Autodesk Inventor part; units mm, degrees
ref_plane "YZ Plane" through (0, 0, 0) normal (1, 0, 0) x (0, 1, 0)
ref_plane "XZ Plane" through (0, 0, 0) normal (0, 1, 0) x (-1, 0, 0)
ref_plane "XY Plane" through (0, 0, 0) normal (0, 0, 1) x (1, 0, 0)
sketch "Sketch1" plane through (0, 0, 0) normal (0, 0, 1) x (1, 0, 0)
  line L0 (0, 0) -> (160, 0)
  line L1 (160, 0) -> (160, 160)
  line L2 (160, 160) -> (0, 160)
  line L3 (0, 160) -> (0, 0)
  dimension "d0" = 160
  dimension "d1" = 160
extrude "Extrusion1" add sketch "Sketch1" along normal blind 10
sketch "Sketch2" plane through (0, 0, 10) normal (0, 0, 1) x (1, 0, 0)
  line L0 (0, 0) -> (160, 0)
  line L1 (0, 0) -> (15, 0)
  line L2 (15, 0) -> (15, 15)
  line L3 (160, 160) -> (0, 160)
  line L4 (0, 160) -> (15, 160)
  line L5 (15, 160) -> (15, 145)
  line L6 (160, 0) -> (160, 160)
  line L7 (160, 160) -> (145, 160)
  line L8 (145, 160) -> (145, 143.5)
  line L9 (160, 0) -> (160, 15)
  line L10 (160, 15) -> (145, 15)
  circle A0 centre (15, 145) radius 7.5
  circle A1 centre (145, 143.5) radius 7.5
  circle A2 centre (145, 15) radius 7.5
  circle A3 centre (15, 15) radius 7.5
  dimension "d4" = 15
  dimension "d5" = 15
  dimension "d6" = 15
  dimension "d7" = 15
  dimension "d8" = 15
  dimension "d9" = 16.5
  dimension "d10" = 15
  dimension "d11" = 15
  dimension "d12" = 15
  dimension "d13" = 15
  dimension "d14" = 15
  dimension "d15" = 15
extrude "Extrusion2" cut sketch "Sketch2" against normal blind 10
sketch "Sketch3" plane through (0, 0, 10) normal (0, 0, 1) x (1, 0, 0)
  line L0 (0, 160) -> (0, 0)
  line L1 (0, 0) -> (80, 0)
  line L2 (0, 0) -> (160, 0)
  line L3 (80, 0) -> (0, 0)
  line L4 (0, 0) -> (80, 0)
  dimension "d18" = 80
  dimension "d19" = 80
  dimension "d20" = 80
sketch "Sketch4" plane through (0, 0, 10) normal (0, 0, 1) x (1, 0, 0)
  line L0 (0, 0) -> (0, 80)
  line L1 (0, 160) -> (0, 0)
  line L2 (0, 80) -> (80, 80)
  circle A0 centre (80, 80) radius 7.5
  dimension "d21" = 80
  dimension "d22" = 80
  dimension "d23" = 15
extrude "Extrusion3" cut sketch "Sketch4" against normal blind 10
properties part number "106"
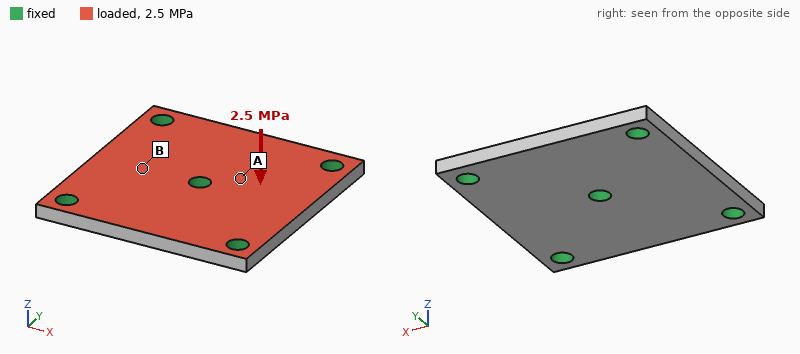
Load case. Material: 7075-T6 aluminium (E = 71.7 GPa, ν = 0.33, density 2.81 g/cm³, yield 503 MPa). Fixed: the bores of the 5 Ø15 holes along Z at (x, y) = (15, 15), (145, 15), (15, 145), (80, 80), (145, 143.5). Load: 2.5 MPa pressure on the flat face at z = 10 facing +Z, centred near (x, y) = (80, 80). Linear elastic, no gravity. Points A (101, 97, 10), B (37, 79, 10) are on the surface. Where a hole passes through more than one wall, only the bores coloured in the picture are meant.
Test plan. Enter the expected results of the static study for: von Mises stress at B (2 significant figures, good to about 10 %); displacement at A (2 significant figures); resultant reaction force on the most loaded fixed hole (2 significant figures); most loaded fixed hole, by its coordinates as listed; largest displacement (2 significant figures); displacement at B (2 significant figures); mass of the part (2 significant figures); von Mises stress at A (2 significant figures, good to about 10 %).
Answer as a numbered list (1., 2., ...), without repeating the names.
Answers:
1. 22 MPa
2. 0.061 mm
3. 21 kN
4. (80, 80)
5. 0.20 mm
6. 0.12 mm
7. 690 g
8. 53 MPa
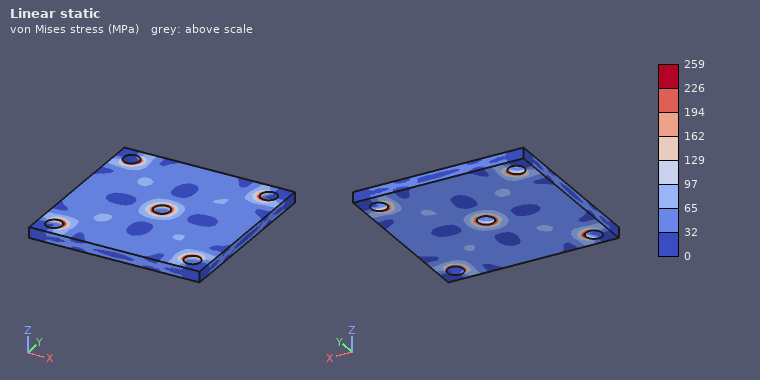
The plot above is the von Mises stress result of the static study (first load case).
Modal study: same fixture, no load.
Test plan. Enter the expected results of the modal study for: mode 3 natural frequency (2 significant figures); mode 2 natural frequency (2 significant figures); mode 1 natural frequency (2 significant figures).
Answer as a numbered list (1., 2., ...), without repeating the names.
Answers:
1. 4100 Hz
2. 4100 Hz
3. 3900 Hz
